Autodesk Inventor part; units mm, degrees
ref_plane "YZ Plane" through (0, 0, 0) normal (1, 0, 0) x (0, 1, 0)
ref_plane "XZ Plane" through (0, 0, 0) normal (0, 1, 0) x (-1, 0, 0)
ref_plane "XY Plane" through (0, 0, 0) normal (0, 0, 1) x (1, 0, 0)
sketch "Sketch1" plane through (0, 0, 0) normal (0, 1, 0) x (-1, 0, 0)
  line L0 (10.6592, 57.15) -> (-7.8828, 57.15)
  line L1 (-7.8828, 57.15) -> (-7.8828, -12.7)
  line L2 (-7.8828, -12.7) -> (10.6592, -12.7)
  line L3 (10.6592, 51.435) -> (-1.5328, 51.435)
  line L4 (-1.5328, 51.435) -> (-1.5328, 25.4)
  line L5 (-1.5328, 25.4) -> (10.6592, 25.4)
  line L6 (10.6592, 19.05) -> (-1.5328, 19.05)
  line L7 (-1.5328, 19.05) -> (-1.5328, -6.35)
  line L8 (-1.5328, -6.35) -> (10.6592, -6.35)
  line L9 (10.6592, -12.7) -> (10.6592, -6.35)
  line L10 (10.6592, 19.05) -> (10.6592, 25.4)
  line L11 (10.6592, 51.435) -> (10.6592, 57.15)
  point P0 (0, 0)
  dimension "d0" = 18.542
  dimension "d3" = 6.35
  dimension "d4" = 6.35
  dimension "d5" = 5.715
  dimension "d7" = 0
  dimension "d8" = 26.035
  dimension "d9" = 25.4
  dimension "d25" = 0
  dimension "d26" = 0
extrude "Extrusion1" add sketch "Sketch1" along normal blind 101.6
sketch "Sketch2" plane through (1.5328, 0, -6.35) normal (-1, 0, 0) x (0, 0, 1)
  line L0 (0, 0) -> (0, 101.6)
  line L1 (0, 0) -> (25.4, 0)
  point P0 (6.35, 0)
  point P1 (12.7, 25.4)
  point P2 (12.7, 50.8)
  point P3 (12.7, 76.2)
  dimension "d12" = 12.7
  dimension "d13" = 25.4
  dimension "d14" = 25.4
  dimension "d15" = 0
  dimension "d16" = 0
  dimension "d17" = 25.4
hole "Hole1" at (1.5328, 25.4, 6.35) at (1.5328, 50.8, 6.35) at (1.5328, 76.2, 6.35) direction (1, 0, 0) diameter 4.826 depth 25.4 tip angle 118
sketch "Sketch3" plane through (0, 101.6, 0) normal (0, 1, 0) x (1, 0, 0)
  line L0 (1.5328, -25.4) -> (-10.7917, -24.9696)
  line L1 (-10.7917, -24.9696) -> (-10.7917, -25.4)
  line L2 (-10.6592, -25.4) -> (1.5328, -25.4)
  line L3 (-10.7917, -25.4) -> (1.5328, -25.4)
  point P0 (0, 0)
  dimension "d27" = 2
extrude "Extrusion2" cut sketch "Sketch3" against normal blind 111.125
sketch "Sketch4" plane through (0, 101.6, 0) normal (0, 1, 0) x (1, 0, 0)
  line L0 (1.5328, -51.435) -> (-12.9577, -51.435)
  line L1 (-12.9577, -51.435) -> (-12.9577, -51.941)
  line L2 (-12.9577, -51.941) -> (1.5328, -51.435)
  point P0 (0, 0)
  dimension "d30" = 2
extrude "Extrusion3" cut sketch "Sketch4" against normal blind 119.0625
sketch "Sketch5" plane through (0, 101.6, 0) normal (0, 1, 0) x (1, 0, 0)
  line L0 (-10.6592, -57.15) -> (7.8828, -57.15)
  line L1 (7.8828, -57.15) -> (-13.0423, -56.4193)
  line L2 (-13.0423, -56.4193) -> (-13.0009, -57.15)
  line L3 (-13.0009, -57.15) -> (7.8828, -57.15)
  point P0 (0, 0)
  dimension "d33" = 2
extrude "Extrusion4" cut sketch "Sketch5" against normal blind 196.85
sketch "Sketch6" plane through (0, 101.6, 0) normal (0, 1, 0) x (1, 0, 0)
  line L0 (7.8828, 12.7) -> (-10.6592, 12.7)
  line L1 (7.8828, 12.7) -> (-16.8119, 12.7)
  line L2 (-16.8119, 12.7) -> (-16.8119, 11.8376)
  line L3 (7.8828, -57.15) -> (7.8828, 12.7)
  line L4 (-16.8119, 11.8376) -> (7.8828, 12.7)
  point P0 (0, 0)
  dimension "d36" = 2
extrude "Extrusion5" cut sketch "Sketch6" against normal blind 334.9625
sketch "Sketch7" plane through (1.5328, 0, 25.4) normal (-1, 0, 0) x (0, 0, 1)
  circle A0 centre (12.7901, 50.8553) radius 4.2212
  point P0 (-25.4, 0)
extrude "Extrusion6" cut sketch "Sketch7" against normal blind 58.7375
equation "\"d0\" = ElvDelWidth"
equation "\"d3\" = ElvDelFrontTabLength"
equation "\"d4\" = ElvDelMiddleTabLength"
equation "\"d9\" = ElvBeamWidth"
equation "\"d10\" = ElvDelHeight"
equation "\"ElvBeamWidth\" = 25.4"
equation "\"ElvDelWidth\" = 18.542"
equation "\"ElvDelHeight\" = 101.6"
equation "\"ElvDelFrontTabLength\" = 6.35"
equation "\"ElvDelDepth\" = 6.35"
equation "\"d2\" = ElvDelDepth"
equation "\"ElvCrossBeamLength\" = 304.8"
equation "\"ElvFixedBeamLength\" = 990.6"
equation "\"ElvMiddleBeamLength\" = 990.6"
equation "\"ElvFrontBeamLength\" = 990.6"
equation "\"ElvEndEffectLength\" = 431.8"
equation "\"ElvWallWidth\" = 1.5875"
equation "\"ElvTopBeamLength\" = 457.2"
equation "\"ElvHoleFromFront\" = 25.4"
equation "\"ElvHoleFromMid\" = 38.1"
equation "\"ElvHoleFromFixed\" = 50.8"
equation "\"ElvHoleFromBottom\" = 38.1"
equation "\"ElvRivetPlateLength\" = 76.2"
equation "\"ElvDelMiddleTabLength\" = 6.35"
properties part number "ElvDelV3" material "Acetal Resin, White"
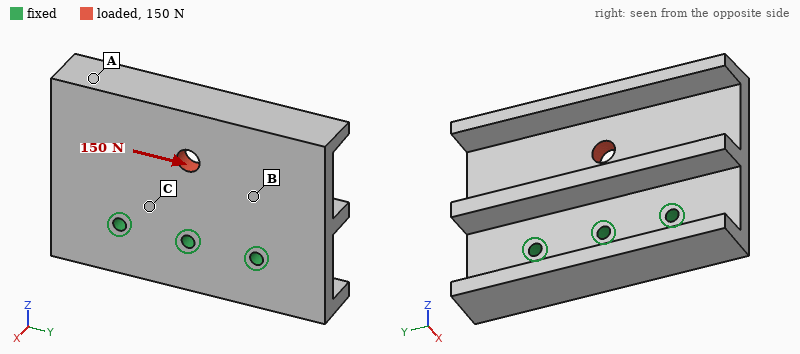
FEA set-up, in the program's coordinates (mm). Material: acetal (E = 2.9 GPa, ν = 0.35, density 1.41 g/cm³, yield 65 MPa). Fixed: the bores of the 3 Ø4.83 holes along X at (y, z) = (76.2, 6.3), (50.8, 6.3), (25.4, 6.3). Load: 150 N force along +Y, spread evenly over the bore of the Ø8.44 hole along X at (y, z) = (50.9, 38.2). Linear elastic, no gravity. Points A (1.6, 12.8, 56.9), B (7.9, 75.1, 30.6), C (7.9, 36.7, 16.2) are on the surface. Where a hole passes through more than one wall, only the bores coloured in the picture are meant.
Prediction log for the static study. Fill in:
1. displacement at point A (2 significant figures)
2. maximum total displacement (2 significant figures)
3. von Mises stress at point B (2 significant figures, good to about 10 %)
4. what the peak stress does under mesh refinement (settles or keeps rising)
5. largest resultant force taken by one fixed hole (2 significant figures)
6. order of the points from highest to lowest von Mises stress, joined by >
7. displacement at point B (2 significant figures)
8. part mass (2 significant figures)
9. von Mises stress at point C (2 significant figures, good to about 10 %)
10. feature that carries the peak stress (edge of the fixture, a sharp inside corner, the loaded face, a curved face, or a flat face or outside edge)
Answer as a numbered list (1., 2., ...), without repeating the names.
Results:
1. 19 µm
2. 21 µm
3. 0.41 MPa
4. keeps rising
5. 100 N
6. C > B > A
7. 10 µm
8. 92 g
9. 0.74 MPa
10. edge of the fixture
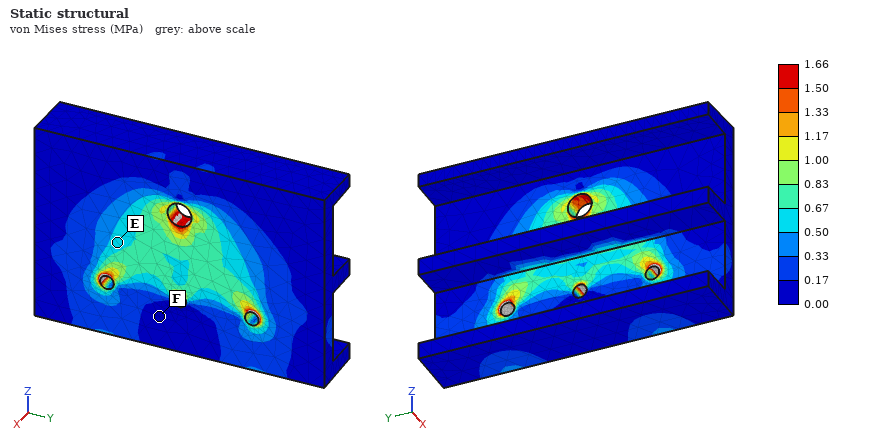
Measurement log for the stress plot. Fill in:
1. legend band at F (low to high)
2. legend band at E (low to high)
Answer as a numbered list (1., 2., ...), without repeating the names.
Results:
1. 0.00 to 0.17 MPa
2. 0.50 to 0.67 MPa
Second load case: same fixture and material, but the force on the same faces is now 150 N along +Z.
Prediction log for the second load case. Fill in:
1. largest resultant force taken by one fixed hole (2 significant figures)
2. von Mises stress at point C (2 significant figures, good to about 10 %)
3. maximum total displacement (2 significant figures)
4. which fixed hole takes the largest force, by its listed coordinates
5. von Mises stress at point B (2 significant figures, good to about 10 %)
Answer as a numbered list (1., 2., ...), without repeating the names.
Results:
1. 63 N
2. 0.33 MPa
3. 9.0 µm
4. (50.8, 6.3)
5. 0.19 MPa
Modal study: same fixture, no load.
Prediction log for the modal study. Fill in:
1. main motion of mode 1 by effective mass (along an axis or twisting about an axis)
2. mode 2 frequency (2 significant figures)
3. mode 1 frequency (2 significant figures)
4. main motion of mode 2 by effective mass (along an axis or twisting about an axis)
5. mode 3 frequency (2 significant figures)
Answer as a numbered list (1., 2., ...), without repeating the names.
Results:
1. along X
2. 640 Hz
3. 420 Hz
4. twisting about Z
5. 1700 Hz
